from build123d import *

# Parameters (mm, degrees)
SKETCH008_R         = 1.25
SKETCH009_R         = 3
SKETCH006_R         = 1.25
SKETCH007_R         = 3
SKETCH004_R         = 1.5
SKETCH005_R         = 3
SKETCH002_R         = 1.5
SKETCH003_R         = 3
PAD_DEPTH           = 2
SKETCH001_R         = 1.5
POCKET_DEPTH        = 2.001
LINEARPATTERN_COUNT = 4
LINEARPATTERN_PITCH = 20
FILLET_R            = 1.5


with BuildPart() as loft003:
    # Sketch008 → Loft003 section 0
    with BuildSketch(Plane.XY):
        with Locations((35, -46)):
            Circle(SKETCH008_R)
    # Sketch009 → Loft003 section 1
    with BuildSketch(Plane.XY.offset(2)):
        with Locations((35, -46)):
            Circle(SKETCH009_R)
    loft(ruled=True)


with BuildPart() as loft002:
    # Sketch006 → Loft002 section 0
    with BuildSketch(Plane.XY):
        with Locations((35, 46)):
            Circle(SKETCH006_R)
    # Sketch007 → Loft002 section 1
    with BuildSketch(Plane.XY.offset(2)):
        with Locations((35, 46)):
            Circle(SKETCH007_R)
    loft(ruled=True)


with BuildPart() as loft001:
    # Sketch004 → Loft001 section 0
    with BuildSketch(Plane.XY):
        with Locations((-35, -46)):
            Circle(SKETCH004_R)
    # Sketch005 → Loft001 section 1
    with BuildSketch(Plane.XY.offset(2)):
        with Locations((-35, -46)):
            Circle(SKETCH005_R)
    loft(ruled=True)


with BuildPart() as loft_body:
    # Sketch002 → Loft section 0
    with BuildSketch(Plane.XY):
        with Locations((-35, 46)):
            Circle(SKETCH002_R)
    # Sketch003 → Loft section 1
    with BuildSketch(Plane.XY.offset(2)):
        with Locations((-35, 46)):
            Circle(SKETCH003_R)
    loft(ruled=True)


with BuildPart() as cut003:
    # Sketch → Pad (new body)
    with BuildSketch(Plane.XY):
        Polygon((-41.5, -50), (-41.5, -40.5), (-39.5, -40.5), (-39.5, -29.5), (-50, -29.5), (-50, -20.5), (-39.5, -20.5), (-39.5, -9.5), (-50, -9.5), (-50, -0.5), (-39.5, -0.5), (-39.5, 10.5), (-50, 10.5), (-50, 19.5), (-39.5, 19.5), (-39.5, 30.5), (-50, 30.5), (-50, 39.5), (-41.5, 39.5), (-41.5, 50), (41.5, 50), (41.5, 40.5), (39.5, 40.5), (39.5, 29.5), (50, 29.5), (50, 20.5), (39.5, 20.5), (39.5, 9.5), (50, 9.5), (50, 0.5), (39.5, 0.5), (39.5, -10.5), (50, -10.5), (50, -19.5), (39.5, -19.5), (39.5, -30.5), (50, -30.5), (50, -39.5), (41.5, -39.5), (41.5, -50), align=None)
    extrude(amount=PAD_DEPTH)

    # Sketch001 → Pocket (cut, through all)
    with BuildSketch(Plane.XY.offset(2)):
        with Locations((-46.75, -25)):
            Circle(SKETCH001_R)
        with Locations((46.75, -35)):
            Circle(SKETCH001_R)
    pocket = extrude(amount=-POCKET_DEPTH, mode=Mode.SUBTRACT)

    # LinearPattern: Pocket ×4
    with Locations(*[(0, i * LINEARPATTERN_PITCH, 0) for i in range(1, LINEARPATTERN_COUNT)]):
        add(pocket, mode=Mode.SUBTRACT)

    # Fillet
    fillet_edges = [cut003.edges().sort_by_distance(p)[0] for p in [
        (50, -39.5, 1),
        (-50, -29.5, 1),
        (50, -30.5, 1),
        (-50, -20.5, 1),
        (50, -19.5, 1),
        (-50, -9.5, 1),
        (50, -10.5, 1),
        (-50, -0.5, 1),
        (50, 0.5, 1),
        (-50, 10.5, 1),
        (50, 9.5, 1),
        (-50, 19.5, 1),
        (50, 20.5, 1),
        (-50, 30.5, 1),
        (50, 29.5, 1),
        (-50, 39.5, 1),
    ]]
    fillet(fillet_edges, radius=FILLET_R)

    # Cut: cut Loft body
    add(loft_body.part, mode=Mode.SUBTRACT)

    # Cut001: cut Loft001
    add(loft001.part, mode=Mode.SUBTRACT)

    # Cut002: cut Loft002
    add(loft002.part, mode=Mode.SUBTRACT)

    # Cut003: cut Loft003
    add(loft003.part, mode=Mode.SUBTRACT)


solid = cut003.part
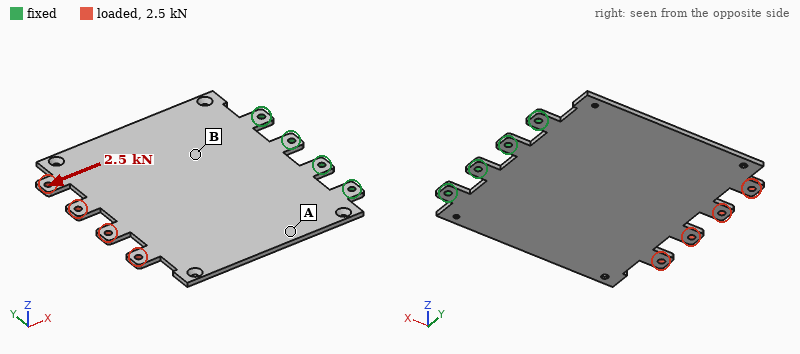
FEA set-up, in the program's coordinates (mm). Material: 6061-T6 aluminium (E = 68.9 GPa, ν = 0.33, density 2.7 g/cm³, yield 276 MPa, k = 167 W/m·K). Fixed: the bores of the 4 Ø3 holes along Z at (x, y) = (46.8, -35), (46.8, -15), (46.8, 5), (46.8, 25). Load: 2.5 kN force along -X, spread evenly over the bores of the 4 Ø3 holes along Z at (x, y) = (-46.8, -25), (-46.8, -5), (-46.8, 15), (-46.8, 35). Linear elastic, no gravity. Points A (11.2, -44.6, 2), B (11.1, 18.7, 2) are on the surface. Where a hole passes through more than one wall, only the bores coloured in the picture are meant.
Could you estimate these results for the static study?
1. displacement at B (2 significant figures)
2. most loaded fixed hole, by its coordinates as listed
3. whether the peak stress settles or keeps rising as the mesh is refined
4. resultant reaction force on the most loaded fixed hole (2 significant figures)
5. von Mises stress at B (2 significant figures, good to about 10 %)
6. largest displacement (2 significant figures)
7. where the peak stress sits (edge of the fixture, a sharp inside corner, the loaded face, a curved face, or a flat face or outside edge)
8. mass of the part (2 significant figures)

18 µm
(46.8, 25)
keeps rising
1.0 kN
20 MPa
44 µm
edge of the fixture
46 g
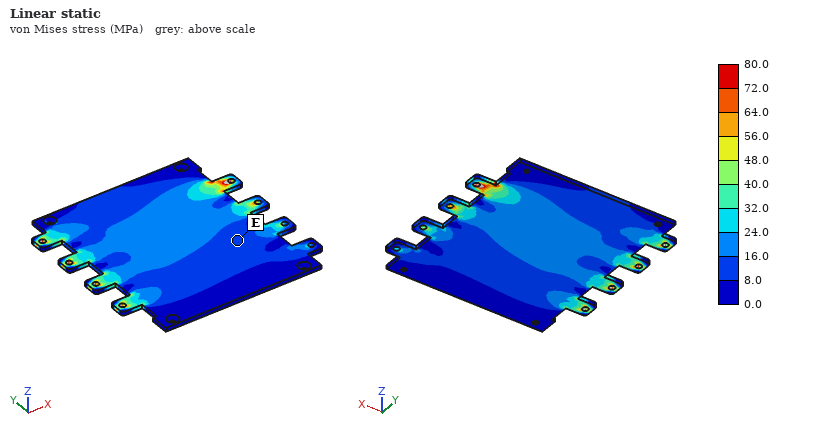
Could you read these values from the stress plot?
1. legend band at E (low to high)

8.0 to 16.0 MPa
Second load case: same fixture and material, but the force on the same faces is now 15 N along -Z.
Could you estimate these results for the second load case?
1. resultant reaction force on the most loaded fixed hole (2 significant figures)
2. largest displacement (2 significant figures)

7.8 N
1.4 mm
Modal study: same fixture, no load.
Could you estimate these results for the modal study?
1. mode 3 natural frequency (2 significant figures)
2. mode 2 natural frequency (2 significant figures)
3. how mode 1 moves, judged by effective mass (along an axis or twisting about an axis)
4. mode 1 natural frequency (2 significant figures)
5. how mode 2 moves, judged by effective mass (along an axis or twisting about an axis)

1000 Hz
400 Hz
along Z
160 Hz
twisting about X
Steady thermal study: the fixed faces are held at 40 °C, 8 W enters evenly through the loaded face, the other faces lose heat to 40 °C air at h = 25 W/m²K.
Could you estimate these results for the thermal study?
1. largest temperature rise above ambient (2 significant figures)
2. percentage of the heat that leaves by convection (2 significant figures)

24 K
51 %
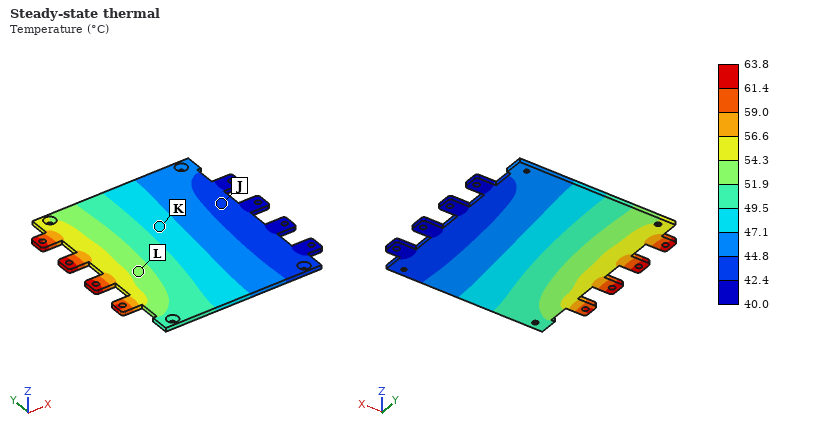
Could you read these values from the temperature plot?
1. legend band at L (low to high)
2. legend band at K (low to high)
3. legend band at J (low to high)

51.9 to 54.3 °C
47.1 to 49.5 °C
42.4 to 44.8 °C
